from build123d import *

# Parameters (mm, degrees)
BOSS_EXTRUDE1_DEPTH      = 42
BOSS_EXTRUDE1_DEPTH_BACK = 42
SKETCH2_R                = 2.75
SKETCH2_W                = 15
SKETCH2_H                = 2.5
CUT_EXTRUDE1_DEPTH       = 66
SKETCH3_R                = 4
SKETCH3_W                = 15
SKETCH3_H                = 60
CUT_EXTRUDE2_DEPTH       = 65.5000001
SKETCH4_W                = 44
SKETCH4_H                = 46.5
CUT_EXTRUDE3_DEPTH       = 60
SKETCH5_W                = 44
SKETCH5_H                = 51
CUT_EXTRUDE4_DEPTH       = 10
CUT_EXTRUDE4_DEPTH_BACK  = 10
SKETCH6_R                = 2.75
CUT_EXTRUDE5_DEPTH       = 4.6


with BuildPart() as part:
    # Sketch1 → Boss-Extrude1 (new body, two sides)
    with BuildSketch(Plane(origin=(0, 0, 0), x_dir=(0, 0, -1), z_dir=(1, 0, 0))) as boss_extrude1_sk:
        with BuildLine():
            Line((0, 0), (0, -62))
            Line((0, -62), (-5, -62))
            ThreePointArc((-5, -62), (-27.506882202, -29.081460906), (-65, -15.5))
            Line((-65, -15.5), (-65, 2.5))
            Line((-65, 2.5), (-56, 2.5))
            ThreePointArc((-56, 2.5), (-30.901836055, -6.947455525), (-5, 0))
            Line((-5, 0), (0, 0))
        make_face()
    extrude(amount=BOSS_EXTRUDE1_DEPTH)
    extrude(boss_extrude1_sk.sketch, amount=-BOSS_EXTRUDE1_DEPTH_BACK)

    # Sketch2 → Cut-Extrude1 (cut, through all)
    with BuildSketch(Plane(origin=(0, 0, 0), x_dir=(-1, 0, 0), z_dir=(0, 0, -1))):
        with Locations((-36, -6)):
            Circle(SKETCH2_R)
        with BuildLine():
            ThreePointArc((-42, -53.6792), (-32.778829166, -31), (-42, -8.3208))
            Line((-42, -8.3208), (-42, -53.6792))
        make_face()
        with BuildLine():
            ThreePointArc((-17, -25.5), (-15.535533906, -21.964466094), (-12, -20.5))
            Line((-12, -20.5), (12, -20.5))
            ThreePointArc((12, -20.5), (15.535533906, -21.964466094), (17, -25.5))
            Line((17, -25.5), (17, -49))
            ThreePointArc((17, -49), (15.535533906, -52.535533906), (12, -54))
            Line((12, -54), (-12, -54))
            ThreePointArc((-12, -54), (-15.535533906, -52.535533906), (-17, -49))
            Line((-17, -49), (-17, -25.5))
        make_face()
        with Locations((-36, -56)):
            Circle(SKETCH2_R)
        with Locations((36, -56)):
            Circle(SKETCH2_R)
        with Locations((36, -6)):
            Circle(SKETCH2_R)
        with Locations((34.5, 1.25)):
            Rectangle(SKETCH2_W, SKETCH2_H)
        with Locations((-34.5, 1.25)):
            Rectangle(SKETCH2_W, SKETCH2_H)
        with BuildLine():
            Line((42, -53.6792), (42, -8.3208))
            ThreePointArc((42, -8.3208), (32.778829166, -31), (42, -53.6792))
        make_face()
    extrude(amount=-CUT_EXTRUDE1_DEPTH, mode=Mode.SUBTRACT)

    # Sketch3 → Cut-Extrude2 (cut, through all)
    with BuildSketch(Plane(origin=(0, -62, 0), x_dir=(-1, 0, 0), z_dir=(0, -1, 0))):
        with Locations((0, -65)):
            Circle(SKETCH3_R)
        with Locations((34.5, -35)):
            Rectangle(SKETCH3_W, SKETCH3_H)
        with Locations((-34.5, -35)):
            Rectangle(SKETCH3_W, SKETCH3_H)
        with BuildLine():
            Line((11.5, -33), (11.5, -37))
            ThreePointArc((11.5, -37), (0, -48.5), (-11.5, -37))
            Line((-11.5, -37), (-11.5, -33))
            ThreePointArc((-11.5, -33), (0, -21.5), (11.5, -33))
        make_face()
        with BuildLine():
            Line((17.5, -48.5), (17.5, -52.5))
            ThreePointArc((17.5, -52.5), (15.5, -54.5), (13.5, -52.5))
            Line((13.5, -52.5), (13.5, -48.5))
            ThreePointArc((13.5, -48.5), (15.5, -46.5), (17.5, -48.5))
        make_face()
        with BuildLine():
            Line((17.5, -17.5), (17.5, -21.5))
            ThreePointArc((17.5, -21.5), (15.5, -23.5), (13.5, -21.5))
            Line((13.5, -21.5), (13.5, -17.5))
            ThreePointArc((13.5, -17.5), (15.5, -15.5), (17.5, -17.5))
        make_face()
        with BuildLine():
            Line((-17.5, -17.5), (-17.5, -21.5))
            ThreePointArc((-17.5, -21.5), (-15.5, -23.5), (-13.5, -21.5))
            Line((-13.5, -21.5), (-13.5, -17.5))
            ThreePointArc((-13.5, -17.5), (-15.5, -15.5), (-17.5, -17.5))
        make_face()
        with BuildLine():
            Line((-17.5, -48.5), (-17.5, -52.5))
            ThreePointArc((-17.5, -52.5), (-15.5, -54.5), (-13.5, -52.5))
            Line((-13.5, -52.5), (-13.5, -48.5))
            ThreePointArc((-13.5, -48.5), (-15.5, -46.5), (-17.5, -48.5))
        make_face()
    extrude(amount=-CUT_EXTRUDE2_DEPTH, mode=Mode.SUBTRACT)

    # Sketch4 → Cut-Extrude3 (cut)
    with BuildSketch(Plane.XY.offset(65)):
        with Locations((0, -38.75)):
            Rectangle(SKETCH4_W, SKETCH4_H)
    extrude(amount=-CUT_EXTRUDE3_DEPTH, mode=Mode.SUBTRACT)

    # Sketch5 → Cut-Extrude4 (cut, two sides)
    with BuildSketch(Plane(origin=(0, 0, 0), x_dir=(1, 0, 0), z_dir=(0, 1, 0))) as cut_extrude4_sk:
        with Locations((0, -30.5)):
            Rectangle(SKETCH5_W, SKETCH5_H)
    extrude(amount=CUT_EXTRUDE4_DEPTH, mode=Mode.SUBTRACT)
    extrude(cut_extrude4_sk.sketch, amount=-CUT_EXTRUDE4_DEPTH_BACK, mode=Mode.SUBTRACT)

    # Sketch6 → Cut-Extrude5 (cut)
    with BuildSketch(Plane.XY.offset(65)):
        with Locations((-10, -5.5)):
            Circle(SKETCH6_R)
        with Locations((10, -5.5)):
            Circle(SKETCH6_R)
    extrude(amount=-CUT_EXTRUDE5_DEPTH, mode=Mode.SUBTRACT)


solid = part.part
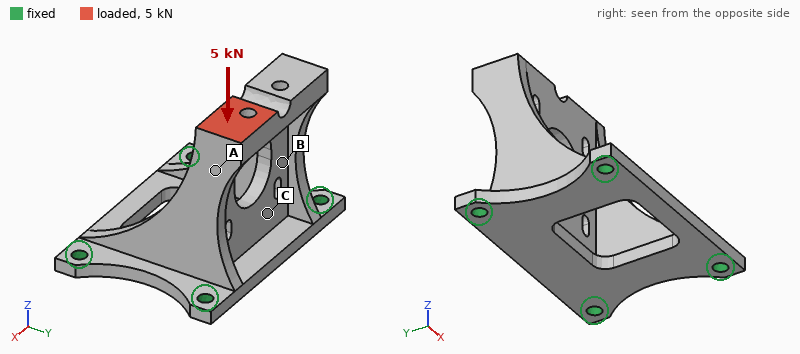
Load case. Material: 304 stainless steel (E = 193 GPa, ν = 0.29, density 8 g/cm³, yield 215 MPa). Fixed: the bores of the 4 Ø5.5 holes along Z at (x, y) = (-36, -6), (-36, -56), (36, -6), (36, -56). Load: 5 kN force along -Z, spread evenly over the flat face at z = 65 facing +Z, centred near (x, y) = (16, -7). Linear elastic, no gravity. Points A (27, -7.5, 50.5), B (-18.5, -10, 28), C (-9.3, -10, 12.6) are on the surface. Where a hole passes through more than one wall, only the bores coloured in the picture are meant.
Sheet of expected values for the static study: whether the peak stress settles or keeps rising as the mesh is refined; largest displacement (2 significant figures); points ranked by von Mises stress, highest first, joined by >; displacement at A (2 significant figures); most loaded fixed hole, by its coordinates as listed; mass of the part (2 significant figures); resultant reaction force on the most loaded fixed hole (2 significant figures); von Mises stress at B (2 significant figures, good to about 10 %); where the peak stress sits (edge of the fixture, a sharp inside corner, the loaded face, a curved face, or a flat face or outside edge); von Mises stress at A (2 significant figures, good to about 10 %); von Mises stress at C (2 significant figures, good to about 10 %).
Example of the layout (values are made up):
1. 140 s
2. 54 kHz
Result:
1. keeps rising
2. 0.11 mm
3. A > B > C
4. 0.063 mm
5. (36, -6)
6. 380 g
7. 3.8 kN
8. 32 MPa
9. edge of the fixture
10. 47 MPa
11. 14 MPa
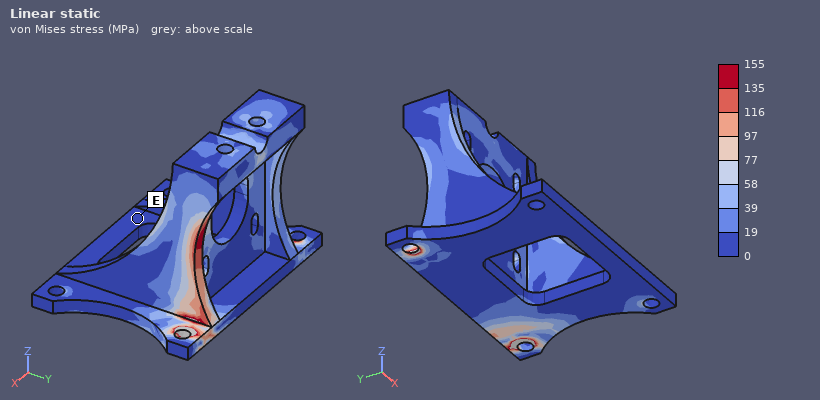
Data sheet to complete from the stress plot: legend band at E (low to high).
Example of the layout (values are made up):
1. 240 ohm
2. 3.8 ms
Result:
1. 0 to 19 MPa
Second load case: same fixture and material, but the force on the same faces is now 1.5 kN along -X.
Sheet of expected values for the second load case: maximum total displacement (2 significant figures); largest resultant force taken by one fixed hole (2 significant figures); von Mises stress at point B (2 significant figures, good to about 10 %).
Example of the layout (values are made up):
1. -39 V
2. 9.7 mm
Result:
1. 29 µm
2. 1.4 kN
3. 22 MPa
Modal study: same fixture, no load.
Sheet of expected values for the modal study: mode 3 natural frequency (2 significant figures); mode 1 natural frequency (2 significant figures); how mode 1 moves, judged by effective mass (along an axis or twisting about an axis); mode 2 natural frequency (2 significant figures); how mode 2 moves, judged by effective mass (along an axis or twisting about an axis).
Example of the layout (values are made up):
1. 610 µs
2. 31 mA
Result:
1. 4300 Hz
2. 2400 Hz
3. along Y
4. 3800 Hz
5. along X
